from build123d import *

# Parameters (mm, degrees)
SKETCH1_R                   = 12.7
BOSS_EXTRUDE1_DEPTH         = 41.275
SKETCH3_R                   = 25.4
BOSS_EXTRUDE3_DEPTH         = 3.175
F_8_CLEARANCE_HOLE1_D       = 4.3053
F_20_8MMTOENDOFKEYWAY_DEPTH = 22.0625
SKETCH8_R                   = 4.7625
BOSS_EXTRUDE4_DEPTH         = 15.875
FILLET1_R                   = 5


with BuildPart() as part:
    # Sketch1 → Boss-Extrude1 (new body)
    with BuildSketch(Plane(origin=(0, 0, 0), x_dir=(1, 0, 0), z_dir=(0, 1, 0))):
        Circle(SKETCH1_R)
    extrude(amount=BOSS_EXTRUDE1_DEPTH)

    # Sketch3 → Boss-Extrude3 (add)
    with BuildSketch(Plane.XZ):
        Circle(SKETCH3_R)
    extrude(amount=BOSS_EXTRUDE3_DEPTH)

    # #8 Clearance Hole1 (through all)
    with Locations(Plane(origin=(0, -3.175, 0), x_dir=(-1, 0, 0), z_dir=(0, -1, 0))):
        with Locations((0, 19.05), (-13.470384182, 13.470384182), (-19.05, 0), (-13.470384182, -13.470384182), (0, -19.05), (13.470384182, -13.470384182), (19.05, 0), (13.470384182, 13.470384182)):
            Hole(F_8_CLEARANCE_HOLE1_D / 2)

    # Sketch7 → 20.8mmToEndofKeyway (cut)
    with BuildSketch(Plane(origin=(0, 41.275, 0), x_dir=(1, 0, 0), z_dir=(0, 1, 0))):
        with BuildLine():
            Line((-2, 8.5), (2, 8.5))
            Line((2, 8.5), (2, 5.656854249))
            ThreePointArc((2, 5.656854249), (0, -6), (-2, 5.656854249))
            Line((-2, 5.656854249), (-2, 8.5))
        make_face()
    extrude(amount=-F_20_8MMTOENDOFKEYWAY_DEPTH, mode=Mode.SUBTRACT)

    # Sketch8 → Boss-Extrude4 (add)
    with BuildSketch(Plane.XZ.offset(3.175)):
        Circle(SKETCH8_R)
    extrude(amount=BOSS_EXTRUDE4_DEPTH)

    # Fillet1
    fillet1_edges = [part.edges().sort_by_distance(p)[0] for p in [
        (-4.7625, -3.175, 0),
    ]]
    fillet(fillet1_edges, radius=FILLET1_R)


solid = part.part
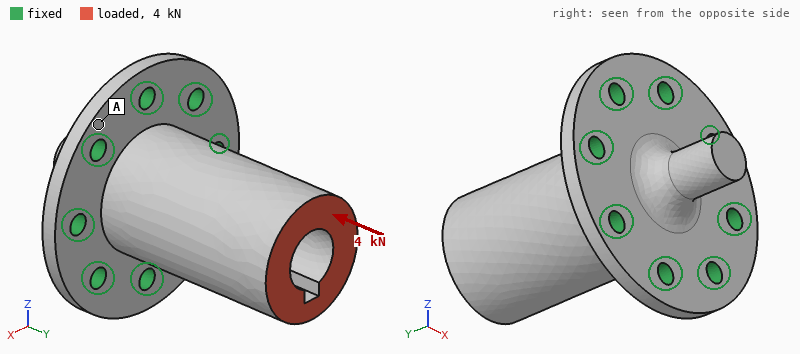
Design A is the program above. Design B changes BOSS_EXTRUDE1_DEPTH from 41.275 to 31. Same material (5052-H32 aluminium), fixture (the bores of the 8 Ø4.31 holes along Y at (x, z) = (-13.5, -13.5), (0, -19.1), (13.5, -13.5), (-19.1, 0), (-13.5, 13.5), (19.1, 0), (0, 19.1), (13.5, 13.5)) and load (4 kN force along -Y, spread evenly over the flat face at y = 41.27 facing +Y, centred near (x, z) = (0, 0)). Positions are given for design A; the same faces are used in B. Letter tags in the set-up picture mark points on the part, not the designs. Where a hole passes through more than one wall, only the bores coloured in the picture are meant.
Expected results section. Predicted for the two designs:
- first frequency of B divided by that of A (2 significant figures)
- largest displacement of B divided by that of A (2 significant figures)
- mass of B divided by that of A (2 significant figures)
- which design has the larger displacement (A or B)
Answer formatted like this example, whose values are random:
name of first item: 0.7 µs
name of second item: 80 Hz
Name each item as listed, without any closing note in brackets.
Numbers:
first frequency of B divided by that of A: 1.5
largest displacement of B divided by that of A: 0.90
mass of B divided by that of A: 0.85
which design has the larger displacement: A
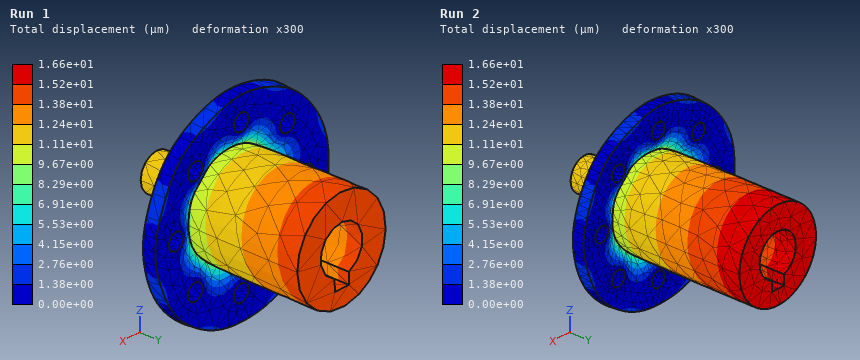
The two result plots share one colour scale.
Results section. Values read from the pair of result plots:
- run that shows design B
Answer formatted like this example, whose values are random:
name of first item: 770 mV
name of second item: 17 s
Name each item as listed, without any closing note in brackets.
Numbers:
run that shows design B: Run 1
